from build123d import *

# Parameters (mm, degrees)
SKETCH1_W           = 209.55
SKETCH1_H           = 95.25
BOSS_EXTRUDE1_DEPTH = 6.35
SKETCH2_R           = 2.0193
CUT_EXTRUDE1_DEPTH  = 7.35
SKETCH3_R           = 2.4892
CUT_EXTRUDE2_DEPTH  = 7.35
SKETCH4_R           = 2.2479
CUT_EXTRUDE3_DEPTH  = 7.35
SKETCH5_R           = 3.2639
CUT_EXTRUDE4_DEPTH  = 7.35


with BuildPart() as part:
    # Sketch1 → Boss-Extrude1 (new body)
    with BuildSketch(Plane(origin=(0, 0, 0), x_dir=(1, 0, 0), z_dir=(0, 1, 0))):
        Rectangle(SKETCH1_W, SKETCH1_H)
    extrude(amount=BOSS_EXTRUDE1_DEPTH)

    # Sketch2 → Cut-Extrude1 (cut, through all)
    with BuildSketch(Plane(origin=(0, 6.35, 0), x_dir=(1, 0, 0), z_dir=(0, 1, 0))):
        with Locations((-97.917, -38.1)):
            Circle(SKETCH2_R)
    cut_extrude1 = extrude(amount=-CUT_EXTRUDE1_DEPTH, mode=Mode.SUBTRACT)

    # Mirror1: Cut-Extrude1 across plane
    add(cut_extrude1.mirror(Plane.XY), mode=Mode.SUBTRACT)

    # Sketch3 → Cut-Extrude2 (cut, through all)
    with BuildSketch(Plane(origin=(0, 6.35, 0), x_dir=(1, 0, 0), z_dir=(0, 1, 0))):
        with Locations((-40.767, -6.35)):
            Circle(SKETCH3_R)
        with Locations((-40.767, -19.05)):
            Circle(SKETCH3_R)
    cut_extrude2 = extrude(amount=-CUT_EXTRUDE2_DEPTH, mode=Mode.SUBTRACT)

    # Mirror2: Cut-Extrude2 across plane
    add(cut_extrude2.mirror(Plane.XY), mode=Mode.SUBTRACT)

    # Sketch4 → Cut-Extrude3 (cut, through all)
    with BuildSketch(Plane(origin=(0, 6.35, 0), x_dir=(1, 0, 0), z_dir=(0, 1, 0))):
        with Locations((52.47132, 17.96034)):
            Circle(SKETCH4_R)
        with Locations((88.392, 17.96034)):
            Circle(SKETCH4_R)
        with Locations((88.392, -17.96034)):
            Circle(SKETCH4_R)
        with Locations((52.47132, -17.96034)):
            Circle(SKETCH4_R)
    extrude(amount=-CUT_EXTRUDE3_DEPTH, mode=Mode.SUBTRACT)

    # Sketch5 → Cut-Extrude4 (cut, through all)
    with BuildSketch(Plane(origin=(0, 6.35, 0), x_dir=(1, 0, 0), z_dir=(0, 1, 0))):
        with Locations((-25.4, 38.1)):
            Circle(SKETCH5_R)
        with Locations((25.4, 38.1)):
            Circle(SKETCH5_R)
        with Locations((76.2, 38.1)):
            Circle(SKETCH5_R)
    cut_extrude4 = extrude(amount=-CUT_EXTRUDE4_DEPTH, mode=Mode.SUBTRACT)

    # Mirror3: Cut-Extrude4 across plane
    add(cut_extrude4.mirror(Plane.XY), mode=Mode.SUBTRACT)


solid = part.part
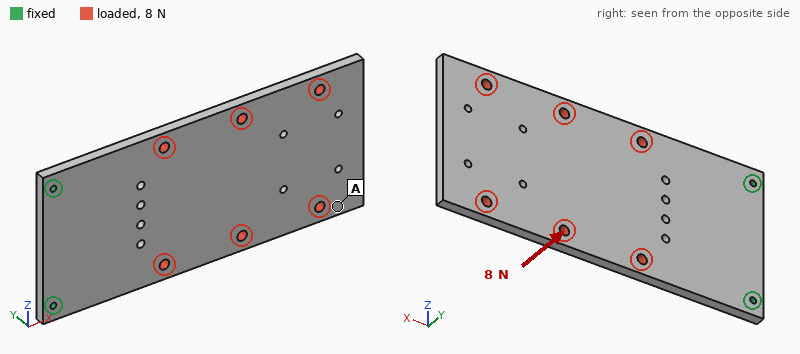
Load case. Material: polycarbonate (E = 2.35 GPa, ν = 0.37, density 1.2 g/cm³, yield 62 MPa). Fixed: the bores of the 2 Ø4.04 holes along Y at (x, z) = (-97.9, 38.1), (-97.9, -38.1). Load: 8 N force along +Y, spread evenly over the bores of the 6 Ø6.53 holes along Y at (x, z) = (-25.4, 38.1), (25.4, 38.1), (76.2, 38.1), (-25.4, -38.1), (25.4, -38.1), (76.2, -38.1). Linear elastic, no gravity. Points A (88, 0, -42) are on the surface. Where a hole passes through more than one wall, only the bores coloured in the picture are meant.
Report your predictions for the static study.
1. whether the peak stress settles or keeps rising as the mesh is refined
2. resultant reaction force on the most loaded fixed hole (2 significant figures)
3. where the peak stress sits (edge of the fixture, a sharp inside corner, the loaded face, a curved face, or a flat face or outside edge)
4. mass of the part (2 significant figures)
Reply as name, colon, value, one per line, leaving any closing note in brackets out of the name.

whether the peak stress settles or keeps rising as the mesh is refined: keeps rising
resultant reaction force on the most loaded fixed hole: 4.0 N
where the peak stress sits: edge of the fixture
mass of the part: 150 g
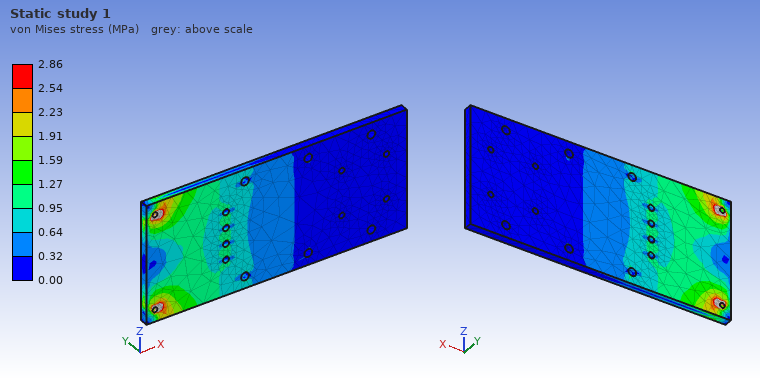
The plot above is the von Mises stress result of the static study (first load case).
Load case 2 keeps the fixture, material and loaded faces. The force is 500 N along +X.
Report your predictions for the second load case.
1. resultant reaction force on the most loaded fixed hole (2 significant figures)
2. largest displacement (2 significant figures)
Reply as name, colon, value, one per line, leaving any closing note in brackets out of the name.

resultant reaction force on the most loaded fixed hole: 260 N
largest displacement: 65 µm
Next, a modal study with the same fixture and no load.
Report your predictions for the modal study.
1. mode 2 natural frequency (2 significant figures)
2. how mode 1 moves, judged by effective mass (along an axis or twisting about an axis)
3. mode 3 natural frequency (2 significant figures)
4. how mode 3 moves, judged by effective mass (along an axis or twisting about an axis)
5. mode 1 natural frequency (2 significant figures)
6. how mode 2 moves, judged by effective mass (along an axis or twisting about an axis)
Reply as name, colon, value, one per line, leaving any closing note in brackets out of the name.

mode 2 natural frequency: 150 Hz
how mode 1 moves, judged by effective mass: along Y
mode 3 natural frequency: 200 Hz
how mode 3 moves, judged by effective mass: along Y
mode 1 natural frequency: 31 Hz
how mode 2 moves, judged by effective mass: twisting about X
